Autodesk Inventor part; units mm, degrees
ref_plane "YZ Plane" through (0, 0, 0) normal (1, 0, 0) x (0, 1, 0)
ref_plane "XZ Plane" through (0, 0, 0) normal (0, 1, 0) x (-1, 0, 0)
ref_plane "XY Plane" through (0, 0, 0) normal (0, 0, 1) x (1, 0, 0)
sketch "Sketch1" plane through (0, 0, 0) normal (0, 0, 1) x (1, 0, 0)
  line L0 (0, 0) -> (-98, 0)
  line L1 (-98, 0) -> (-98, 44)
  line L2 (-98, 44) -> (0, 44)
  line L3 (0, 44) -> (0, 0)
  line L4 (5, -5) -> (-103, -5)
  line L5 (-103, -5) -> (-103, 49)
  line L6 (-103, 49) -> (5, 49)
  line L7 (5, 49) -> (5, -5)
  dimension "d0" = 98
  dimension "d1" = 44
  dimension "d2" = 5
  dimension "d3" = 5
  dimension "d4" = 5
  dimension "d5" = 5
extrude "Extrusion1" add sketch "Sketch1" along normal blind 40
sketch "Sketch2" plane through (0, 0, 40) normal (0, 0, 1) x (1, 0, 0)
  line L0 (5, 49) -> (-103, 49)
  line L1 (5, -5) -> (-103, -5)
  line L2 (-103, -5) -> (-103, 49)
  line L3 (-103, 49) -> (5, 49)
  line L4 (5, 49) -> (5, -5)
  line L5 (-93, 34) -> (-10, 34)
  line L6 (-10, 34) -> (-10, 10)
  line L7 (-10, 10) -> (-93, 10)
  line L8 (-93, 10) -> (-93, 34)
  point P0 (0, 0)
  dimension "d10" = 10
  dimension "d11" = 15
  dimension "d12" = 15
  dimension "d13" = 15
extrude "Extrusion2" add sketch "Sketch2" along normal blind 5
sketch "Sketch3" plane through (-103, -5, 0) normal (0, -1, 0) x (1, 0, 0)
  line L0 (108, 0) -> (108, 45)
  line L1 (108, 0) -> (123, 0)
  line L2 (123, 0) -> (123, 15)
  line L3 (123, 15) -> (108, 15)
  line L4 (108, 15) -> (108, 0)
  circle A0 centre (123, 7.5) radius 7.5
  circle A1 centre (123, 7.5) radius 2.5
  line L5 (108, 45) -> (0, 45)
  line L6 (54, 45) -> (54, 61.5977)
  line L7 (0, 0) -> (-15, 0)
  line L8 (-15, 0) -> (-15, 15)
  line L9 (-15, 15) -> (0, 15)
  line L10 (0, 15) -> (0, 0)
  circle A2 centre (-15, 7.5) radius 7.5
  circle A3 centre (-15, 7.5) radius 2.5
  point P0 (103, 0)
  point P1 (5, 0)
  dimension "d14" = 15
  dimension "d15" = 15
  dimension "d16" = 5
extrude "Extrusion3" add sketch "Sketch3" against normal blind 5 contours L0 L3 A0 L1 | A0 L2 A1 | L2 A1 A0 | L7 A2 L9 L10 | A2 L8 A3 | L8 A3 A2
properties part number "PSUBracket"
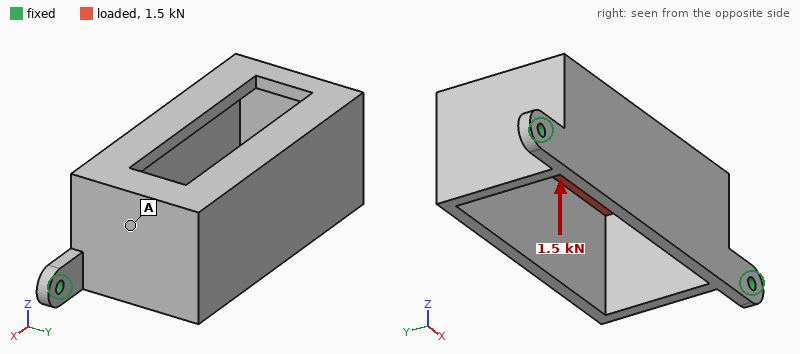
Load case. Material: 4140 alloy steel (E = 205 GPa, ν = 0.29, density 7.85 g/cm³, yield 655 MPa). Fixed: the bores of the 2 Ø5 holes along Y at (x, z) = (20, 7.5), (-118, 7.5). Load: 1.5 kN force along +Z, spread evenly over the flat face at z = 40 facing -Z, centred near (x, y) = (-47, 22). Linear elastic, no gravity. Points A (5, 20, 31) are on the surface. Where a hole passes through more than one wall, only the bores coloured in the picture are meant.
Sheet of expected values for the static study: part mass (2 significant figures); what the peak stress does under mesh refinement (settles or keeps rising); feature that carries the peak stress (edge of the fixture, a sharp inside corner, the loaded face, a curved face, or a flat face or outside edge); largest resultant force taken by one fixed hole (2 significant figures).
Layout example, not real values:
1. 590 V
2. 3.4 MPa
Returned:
1. 650 g
2. keeps rising
3. edge of the fixture
4. 830 N
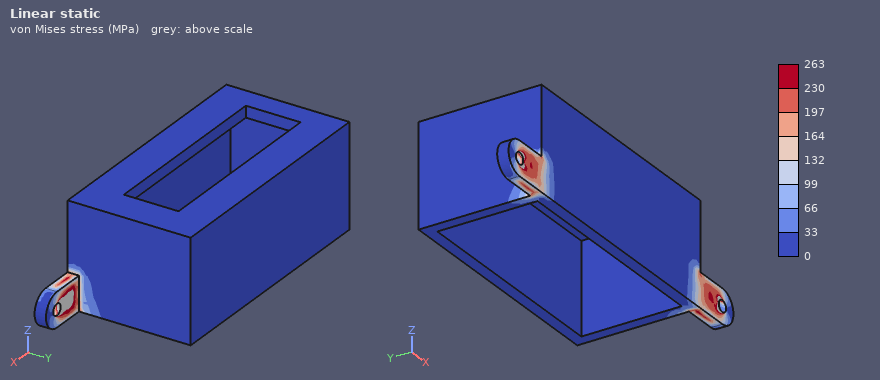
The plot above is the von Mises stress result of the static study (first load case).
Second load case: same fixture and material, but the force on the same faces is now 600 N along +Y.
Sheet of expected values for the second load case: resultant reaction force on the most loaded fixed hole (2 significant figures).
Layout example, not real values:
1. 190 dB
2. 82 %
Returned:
1. 320 N
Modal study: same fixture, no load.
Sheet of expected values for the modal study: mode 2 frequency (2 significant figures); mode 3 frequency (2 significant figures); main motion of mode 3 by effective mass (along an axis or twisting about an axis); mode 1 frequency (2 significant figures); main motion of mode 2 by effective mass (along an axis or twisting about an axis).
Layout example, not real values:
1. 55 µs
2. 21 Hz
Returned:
1. 1000 Hz
2. 1700 Hz
3. along Y
4. 390 Hz
5. along X
